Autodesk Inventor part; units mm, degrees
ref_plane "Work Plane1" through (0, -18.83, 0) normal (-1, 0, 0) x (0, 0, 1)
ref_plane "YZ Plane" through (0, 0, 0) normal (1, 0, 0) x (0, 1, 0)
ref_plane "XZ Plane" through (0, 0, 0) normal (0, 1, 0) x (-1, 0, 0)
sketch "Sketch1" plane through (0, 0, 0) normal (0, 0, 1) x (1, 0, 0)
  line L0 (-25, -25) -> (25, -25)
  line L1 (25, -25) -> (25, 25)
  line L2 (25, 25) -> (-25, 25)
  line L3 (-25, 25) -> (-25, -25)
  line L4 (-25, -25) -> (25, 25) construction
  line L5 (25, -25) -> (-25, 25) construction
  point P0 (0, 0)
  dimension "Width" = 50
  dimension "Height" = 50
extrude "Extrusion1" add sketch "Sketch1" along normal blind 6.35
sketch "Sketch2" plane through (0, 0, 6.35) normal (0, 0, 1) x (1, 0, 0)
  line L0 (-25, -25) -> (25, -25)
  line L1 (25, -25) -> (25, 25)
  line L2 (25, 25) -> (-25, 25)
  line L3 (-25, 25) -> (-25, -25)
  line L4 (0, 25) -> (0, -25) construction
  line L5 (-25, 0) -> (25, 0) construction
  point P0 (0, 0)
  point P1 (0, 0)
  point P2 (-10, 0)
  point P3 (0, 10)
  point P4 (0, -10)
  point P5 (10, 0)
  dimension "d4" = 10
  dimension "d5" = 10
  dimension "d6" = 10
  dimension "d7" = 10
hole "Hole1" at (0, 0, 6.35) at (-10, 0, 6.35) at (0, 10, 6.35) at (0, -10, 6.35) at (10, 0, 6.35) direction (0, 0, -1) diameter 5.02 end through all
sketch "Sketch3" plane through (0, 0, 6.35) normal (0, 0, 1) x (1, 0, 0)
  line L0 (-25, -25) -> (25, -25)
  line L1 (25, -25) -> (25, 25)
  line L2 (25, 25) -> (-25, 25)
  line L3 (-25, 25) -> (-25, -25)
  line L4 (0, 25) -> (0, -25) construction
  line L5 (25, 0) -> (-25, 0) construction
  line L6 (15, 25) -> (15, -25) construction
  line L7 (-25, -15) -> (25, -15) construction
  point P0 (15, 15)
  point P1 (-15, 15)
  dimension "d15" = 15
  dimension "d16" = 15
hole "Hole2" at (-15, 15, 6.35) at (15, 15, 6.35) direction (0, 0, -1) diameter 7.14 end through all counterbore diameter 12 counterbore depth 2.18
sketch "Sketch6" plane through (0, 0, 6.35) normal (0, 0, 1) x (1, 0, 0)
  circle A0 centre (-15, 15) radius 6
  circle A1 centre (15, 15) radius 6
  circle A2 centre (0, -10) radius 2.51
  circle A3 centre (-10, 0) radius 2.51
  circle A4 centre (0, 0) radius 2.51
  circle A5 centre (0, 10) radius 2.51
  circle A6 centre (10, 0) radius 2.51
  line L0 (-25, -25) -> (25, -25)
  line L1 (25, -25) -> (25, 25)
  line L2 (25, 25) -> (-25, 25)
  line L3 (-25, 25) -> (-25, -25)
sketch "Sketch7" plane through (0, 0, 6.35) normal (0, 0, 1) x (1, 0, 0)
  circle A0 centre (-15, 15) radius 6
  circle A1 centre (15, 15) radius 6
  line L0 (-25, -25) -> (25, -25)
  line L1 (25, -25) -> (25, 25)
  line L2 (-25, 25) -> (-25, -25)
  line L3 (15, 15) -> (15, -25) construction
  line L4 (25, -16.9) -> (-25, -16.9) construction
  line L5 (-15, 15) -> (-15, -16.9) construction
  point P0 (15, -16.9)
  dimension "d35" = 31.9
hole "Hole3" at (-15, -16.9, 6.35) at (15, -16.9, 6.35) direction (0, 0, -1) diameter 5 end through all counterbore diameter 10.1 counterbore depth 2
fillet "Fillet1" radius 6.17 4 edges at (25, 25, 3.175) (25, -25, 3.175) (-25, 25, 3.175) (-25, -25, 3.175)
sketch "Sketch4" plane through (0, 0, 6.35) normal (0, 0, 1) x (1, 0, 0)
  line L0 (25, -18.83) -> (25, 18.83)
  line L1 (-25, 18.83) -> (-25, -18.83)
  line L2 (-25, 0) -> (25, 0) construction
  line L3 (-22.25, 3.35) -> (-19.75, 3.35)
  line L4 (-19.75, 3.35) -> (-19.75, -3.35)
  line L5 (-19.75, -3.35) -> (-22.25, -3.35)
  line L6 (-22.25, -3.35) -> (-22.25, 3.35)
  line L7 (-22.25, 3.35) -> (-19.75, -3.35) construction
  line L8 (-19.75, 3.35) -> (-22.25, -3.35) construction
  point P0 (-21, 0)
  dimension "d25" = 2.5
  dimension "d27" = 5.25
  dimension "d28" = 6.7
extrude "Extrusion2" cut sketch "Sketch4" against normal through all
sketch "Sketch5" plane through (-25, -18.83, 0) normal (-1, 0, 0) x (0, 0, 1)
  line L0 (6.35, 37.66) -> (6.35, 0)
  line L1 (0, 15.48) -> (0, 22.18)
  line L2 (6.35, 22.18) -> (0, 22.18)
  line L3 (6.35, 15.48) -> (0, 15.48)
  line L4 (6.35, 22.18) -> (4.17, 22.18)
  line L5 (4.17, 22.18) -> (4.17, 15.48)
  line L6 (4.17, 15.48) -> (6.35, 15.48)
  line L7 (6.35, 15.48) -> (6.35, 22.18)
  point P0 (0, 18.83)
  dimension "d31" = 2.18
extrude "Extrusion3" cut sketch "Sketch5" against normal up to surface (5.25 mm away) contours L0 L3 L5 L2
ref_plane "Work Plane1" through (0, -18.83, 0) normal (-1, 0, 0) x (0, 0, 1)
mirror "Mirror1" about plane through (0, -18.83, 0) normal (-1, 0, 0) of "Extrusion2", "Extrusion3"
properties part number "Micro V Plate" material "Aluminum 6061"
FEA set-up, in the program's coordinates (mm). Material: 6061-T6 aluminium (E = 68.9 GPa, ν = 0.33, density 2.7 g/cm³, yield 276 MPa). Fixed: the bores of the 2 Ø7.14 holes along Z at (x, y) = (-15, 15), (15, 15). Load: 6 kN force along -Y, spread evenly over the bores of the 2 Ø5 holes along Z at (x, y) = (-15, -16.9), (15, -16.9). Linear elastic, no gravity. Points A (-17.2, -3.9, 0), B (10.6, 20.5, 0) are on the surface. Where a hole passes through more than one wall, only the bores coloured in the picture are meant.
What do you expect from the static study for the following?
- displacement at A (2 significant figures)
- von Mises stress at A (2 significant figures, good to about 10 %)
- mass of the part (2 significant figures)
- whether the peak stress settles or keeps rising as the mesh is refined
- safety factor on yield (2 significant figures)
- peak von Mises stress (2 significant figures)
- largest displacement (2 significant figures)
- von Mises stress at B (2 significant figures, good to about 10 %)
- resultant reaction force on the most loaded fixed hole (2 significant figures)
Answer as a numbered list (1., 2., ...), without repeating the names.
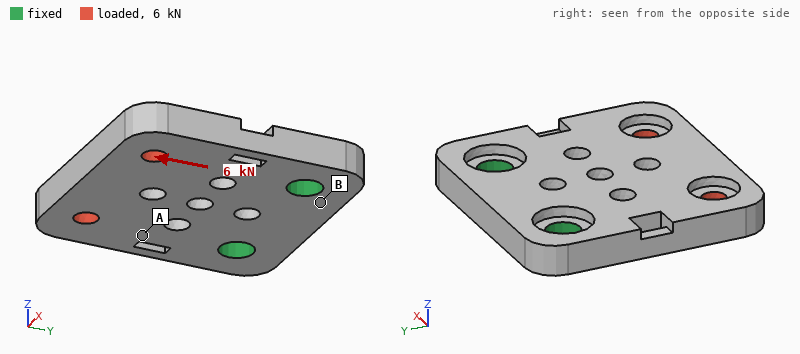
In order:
1. 15 µm
2. 53 MPa
3. 36 g
4. settles
5. 2.7
6. 100 MPa
7. 57 µm
8. 15 MPa
9. 3.0 kN
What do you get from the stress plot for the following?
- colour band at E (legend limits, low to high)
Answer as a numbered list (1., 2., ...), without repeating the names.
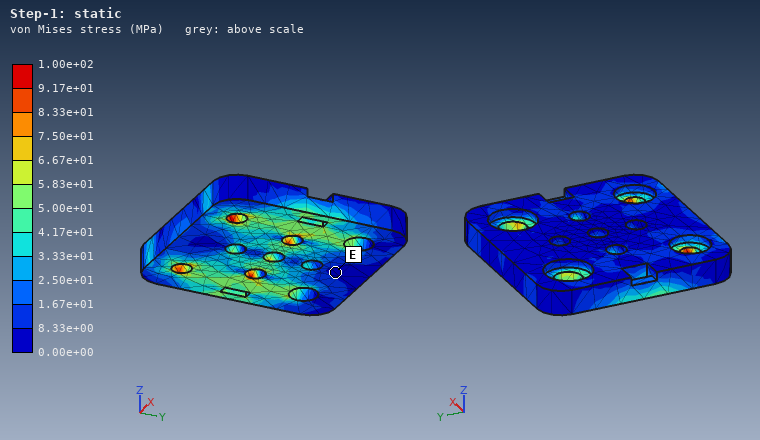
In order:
1. 0.00e+00 to 8.33e+00 MPa
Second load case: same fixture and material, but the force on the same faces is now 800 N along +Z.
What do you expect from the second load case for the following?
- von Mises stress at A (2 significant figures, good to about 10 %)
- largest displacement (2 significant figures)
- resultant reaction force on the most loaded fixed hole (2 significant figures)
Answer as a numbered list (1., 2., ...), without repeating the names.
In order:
1. 42 MPa
2. 0.25 mm
3. 410 N
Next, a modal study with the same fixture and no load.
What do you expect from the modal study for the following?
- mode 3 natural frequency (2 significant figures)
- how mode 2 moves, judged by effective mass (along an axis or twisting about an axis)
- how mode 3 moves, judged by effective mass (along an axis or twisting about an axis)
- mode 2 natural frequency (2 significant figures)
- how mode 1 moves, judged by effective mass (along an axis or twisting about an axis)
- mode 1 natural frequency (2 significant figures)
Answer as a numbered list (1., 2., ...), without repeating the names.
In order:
1. 12 kHz
2. twisting about Y
3. along X
4. 5800 Hz
5. along Z
6. 2800 Hz
